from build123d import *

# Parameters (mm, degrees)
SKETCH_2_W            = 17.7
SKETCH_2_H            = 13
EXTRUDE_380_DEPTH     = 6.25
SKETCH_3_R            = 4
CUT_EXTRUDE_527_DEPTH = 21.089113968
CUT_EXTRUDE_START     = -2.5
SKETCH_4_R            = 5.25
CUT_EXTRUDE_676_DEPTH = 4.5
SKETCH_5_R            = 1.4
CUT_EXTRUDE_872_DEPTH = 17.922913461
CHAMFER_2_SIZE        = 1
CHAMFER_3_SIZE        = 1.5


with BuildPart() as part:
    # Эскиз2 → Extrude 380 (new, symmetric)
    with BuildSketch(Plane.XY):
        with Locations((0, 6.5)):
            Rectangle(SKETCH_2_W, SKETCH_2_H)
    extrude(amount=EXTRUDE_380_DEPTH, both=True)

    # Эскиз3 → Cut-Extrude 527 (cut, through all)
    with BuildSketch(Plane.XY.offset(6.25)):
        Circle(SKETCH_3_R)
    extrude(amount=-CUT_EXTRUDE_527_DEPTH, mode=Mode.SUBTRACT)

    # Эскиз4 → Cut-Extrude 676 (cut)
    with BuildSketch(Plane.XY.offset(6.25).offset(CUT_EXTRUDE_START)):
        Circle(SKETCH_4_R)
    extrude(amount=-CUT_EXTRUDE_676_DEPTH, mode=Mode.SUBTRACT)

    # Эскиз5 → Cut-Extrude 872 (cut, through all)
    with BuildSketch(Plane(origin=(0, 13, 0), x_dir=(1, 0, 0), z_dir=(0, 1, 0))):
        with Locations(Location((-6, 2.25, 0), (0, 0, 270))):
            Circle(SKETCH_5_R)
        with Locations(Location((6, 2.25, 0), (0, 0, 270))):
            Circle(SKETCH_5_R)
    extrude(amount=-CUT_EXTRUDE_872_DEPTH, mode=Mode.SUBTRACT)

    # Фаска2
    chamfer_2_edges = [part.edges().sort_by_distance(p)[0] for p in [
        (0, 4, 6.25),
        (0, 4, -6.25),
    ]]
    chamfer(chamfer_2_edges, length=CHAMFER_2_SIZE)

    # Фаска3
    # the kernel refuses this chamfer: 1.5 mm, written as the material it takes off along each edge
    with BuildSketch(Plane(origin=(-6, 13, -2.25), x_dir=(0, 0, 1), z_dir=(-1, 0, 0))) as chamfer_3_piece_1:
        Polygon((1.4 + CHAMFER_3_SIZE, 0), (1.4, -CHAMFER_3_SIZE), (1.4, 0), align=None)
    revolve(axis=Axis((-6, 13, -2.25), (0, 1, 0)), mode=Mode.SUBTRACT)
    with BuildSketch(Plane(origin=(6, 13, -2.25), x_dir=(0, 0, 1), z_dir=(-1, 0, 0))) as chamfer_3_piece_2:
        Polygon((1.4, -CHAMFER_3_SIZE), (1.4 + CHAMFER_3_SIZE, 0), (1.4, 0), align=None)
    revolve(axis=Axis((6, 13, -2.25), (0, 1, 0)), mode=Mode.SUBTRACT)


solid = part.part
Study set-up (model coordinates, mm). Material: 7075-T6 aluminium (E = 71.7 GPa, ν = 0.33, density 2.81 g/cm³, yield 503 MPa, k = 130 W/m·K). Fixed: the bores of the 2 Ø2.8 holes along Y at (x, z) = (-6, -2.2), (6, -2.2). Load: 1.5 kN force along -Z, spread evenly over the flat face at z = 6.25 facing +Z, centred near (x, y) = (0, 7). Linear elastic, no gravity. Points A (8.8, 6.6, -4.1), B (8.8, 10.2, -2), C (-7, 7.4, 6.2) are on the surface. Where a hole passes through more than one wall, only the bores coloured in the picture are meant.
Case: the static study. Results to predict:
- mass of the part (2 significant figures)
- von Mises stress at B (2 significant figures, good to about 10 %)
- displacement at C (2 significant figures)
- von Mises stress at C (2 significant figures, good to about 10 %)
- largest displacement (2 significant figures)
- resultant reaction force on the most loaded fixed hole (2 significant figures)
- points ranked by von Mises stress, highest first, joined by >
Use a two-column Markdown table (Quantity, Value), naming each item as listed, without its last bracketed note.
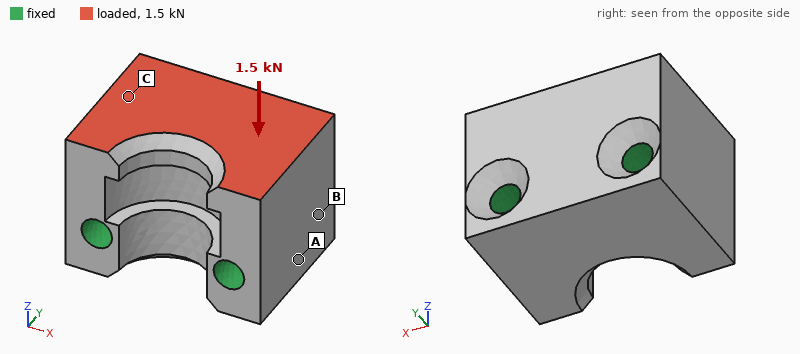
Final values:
| Quantity | Value |
|---|---|
| mass of the part | 6.4 g |
| von Mises stress at B | 6.3 MPa |
| displacement at C | 1.0 µm |
| von Mises stress at C | 8.7 MPa |
| largest displacement | 1.5 µm |
| resultant reaction force on the most loaded fixed hole | 760 N |
| points ranked by von Mises stress, highest first, joined by > | C > B > A |
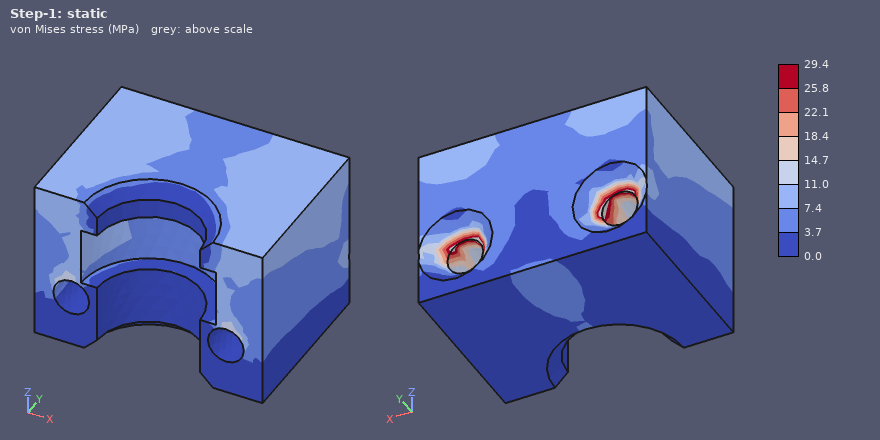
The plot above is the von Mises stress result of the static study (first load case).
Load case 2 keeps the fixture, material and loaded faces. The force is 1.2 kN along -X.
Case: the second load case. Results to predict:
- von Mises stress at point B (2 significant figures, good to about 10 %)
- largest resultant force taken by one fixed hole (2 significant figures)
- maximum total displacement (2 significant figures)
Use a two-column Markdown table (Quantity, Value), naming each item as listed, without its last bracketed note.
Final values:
| Quantity | Value |
|---|---|
| von Mises stress at point B | 16 MPa |
| largest resultant force taken by one fixed hole | 890 N |
| maximum total displacement | 5.6 µm |
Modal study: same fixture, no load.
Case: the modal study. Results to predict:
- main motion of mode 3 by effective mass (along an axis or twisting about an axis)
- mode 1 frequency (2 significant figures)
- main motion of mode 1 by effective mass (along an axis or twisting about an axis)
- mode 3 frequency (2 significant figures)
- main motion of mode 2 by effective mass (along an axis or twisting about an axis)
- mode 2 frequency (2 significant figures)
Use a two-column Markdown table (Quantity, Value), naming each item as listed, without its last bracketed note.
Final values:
| Quantity | Value |
|---|---|
| main motion of mode 3 by effective mass | along X |
| mode 1 frequency | 63 kHz |
| main motion of mode 1 by effective mass | along Y |
| mode 3 frequency | 83 kHz |
| main motion of mode 2 by effective mass | along X |
| mode 2 frequency | 67 kHz |
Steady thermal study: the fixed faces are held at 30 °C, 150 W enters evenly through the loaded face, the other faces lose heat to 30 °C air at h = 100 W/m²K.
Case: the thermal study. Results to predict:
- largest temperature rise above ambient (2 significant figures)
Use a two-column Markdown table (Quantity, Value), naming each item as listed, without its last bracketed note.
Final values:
| Quantity | Value |
|---|---|
| largest temperature rise above ambient | 53 K |
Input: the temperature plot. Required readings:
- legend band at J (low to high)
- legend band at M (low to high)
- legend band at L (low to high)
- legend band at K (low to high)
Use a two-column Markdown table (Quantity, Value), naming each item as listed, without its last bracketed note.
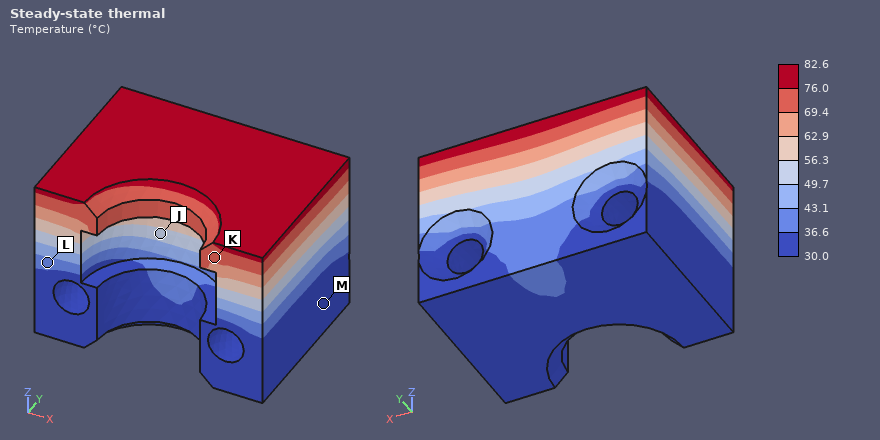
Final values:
| Quantity | Value |
|---|---|
| legend band at J | 49.7 to 56.3 °C |
| legend band at M | 30.0 to 36.6 °C |
| legend band at L | 36.6 to 43.1 °C |
| legend band at K | 69.4 to 76.0 °C |
